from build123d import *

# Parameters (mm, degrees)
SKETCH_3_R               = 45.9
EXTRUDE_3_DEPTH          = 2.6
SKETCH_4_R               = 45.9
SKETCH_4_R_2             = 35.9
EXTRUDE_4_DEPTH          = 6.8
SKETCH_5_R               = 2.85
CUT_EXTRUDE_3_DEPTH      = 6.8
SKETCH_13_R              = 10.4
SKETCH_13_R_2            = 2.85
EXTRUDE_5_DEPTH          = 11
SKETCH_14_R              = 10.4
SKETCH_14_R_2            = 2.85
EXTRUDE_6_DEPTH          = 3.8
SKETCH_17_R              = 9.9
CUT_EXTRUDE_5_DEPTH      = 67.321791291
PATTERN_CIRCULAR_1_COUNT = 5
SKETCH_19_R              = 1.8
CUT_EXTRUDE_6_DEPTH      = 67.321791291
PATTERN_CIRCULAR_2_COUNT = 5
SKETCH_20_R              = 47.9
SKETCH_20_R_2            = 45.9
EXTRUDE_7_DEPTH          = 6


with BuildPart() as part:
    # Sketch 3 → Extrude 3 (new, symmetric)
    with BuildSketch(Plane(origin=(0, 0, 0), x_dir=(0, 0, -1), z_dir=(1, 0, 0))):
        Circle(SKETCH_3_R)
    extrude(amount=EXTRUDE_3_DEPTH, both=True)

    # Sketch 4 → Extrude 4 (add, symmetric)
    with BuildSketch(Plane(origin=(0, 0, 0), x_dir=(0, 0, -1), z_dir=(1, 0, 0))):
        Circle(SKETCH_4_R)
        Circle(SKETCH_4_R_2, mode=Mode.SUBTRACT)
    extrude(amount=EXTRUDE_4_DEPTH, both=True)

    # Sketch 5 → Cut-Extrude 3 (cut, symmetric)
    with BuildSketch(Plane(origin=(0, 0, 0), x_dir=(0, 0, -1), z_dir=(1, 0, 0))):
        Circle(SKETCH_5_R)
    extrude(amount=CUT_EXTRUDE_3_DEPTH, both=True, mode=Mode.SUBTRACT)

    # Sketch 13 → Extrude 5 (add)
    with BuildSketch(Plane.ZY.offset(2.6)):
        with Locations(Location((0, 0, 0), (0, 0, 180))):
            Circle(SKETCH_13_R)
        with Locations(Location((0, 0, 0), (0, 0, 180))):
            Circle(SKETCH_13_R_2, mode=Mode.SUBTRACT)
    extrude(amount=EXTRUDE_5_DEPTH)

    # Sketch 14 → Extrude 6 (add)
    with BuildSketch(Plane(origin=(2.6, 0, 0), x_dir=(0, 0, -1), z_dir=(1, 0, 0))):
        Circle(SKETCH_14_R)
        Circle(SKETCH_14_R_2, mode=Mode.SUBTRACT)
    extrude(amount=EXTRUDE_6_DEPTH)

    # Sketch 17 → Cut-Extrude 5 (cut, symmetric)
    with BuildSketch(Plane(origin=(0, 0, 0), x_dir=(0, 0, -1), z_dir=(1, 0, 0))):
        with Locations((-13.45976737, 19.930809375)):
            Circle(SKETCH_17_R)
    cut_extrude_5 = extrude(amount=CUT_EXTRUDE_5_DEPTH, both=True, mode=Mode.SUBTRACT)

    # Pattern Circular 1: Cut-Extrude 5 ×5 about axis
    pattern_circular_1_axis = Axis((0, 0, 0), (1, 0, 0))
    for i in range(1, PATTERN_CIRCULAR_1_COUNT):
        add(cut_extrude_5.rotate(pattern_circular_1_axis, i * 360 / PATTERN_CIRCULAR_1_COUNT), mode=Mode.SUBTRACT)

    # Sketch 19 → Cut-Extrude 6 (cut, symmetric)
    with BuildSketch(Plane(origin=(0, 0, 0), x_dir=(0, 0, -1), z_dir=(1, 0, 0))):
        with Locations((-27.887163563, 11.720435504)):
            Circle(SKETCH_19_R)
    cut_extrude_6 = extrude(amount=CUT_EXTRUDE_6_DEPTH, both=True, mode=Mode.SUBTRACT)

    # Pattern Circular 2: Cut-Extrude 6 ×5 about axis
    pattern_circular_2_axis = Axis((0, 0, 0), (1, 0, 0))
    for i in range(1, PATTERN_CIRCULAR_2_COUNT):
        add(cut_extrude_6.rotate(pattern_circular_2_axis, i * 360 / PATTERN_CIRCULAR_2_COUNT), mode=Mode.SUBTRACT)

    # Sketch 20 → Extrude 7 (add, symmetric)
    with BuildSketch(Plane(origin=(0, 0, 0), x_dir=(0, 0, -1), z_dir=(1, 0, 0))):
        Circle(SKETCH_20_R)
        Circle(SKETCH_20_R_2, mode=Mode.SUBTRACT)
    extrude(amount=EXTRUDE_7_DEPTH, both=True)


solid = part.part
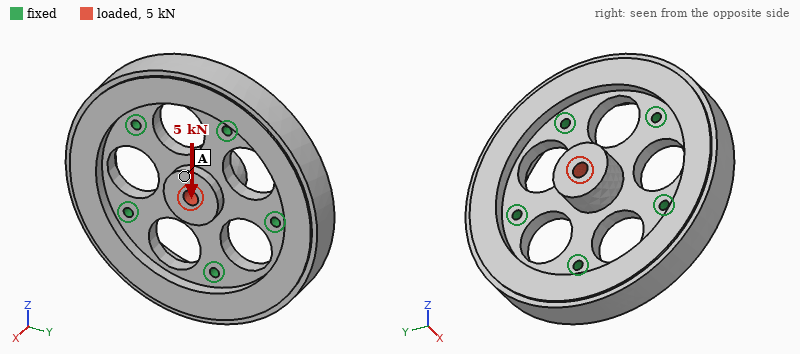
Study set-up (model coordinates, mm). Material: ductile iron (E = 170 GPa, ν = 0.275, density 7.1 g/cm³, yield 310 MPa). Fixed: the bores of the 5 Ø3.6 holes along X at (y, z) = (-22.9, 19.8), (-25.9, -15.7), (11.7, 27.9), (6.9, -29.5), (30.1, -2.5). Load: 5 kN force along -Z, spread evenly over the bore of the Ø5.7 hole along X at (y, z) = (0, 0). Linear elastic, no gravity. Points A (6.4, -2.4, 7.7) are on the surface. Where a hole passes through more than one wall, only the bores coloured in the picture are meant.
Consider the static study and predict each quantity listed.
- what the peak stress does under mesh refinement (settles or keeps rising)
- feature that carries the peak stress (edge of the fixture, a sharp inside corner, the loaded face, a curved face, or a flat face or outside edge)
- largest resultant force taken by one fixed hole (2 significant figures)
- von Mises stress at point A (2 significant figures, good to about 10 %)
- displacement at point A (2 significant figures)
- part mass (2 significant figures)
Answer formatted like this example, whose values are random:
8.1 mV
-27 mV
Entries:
keeps rising
edge of the fixture
1.6 kN
12 MPa
4.6 µm
420 g
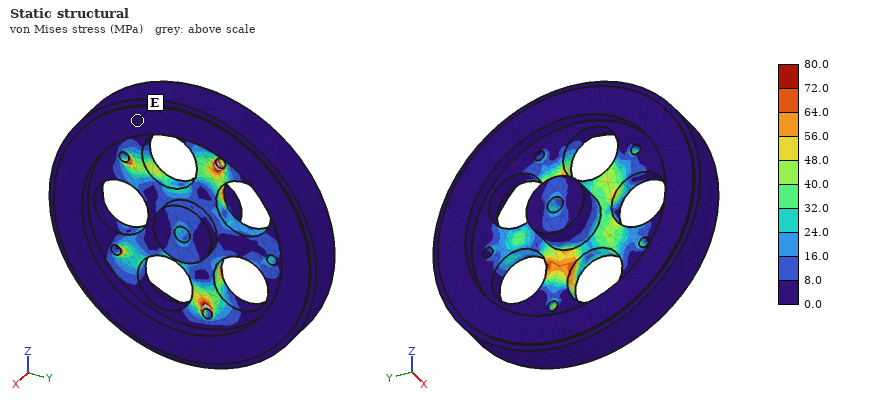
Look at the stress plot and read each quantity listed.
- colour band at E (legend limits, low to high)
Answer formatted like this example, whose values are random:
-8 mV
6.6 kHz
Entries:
0.0 to 8.0 MPa
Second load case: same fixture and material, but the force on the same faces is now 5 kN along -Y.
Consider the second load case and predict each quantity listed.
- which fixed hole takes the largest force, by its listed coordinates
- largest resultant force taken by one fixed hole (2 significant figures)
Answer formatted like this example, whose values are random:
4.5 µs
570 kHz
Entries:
(30.1, -2.5)
1.6 kN
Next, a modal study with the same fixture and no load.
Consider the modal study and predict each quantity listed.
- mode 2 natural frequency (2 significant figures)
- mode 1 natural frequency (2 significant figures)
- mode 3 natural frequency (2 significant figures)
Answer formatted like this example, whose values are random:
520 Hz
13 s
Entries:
6800 Hz
6800 Hz
7000 Hz
